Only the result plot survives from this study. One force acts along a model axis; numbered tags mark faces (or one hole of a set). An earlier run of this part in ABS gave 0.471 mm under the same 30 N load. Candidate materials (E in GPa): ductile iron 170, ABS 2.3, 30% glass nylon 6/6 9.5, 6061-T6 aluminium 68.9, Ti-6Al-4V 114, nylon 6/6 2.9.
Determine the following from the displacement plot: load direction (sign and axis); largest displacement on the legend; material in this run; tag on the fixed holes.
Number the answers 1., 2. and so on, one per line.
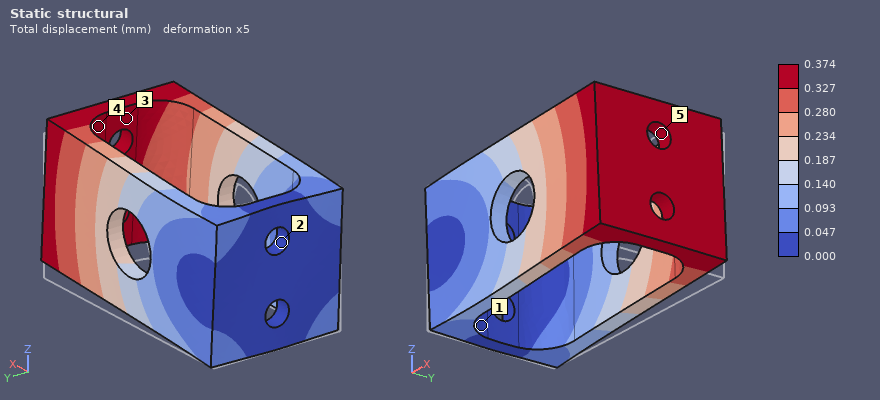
1. +Z
2. 0.374 mm
3. nylon 6/6
4. 2
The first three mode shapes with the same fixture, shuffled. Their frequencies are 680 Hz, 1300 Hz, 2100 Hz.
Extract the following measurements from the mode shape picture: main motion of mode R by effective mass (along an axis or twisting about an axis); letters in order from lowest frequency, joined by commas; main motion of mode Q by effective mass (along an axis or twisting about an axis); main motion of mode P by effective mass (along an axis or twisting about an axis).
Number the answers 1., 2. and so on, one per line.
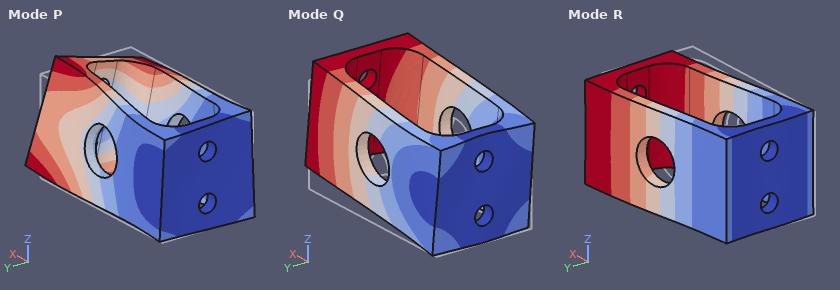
1. along Y
2. R, Q, P
3. along Z
4. twisting about X
